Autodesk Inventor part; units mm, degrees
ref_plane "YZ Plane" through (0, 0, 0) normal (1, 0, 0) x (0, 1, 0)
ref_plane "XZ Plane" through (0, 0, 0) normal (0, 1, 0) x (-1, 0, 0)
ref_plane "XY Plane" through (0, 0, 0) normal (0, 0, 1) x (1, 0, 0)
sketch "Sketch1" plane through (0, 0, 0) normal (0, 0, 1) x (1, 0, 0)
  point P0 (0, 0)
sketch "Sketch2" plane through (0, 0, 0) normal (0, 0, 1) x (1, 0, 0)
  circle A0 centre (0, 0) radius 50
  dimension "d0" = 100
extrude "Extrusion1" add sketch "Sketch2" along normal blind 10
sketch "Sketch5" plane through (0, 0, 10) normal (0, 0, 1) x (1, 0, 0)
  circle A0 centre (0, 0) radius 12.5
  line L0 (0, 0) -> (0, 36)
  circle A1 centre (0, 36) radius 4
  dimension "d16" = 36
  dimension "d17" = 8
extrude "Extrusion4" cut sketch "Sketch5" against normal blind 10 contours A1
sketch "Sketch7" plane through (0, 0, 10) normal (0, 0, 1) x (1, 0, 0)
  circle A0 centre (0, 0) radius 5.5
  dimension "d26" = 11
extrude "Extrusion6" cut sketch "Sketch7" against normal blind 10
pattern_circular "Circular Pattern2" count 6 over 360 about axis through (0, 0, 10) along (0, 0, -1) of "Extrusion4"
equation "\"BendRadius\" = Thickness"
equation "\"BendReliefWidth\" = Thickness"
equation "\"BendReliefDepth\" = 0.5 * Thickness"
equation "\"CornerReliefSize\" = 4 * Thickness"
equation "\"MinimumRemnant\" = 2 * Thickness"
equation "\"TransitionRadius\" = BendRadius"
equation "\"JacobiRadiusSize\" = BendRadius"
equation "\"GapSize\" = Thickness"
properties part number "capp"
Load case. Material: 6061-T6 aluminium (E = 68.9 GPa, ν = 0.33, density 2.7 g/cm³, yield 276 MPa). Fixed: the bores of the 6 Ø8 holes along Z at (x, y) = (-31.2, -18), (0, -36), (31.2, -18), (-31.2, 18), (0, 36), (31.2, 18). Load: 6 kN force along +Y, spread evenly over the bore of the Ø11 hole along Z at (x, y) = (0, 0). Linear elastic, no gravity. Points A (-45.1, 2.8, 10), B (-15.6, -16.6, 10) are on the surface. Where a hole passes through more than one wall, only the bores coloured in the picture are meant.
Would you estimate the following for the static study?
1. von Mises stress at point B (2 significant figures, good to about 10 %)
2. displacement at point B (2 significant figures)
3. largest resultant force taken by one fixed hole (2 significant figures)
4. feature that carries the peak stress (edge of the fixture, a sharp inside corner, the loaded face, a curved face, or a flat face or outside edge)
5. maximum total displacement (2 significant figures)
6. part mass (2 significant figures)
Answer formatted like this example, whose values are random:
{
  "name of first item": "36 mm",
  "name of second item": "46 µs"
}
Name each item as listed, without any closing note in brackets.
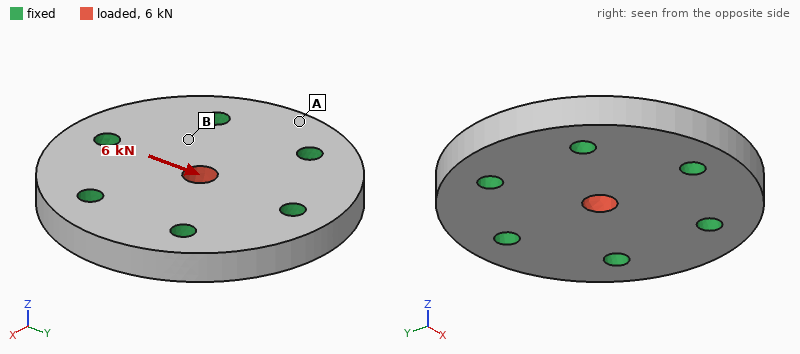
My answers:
{
  "von Mises stress at point B": "4.5 MPa",
  "displacement at point B": "1.4 µm",
  "largest resultant force taken by one fixed hole": "1.6 kN",
  "feature that carries the peak stress": "the loaded face",
  "maximum total displacement": "4.6 µm",
  "part mass": "200 g"
}
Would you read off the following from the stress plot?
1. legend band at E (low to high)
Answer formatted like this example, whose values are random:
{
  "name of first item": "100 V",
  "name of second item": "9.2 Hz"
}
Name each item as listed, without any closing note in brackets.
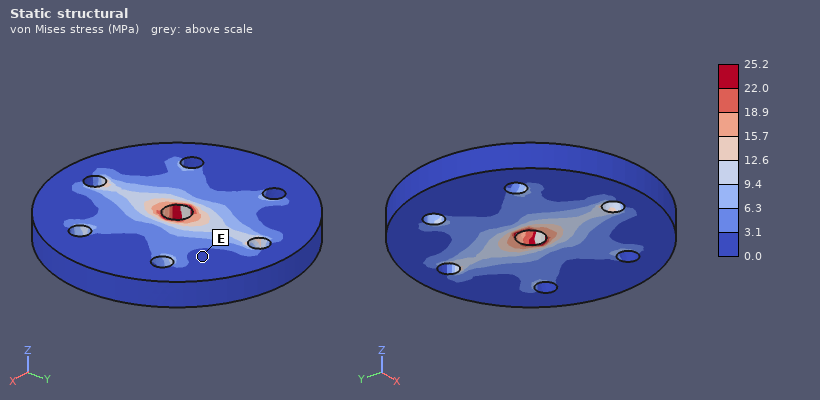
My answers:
{
  "legend band at E": "0.0 to 3.1 MPa"
}
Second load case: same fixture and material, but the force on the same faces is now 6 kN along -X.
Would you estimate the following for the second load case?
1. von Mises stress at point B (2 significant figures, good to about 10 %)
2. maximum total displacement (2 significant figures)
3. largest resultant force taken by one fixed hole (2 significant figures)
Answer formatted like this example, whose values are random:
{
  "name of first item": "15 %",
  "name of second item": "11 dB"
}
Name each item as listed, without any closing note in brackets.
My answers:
{
  "von Mises stress at point B": "5.8 MPa",
  "maximum total displacement": "4.6 µm",
  "largest resultant force taken by one fixed hole": "1.4 kN"
}
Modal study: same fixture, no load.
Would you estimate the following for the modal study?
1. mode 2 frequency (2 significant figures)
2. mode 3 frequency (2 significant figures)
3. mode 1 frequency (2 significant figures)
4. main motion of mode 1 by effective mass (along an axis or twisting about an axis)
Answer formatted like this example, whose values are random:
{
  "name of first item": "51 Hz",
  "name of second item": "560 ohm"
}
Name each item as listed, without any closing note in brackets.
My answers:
{
  "mode 2 frequency": "21 kHz",
  "mode 3 frequency": "21 kHz",
  "mode 1 frequency": "15 kHz",
  "main motion of mode 1 by effective mass": "along Z"
}
